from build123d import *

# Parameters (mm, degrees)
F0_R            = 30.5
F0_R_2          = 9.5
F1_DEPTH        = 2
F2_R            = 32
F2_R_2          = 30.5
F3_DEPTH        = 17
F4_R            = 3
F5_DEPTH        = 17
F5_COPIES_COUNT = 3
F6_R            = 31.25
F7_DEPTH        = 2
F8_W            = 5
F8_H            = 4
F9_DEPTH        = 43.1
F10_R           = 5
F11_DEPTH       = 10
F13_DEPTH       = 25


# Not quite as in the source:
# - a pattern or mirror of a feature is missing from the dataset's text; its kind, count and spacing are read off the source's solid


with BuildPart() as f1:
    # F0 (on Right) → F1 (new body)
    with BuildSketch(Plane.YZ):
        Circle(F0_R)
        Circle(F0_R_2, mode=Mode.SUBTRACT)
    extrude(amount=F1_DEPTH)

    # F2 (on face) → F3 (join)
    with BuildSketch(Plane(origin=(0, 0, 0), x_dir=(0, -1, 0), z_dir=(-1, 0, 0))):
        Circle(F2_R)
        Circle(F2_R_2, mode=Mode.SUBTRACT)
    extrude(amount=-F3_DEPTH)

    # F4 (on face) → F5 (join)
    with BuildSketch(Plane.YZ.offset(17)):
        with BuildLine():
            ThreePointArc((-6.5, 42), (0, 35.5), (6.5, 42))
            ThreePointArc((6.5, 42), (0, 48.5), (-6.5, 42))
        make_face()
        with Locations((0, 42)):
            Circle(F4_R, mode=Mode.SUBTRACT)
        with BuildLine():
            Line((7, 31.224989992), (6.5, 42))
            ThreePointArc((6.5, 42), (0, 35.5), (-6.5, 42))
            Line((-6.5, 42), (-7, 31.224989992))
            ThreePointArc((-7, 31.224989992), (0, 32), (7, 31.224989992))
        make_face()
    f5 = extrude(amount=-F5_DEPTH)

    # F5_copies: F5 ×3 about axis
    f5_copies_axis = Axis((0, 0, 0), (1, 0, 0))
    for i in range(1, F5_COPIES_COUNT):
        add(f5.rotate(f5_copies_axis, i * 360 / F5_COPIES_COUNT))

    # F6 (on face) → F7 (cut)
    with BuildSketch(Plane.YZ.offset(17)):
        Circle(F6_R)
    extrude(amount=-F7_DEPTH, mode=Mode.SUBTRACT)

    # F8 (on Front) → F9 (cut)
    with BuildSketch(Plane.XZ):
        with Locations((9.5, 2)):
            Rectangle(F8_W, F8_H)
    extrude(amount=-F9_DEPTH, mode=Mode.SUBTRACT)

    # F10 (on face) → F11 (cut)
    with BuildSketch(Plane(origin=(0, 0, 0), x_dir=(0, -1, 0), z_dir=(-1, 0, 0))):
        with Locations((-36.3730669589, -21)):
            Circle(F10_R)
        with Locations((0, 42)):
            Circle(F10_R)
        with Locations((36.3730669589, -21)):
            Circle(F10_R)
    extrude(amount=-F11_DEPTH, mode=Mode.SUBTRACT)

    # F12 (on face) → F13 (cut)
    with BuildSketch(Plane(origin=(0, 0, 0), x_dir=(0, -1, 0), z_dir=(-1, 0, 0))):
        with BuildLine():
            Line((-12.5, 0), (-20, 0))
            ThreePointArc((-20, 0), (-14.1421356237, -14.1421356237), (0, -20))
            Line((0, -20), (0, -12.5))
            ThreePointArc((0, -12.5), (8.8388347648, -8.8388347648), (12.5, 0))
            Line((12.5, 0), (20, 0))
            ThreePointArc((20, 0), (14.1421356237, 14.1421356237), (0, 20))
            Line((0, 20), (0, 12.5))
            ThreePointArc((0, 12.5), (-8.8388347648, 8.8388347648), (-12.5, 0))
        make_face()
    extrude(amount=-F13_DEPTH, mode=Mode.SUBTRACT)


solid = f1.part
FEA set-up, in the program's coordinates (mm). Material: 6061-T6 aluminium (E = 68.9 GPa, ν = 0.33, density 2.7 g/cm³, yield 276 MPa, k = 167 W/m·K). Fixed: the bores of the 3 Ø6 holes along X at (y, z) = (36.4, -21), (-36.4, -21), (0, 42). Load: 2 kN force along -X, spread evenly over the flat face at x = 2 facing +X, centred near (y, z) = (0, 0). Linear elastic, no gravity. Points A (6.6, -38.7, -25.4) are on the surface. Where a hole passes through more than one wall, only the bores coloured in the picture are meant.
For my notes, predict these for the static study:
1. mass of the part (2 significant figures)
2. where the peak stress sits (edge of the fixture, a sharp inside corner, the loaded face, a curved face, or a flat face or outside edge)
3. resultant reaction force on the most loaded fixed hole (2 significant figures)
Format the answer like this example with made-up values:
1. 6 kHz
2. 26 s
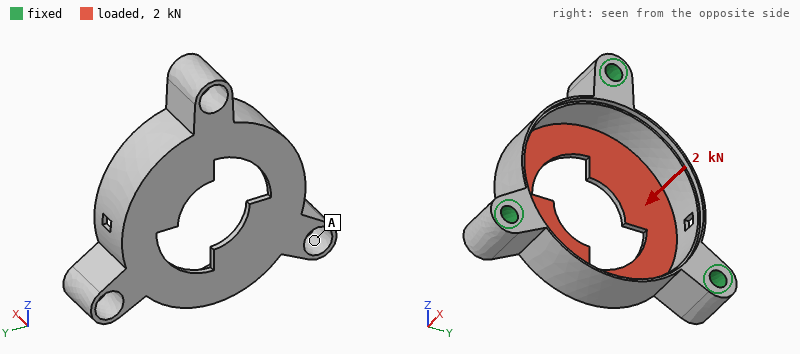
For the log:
1. 44 g
2. a flat face or outside edge
3. 800 N
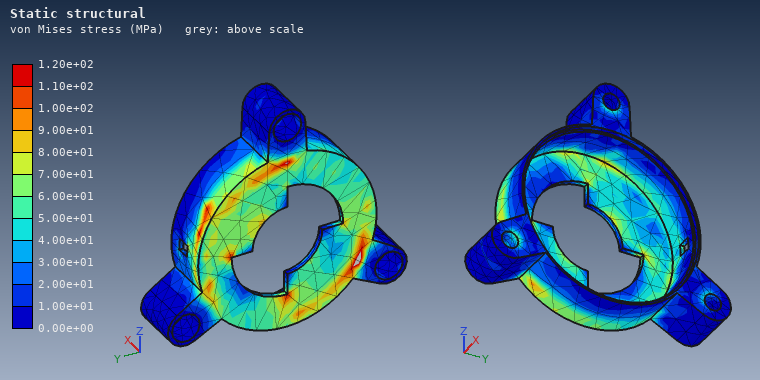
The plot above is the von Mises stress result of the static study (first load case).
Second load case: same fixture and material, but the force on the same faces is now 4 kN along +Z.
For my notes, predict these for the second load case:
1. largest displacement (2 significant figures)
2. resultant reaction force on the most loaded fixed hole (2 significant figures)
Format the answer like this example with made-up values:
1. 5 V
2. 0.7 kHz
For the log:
1. 67 µm
2. 1.5 kN
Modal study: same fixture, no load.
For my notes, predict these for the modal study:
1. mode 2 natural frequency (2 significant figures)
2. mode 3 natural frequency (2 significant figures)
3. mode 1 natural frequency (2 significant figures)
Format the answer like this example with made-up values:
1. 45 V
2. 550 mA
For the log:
1. 6500 Hz
2. 9100 Hz
3. 6200 Hz
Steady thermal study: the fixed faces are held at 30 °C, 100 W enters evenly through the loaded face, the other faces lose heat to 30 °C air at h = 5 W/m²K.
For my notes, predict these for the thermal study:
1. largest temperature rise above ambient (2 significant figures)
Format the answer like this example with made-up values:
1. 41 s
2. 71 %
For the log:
1. 59 K
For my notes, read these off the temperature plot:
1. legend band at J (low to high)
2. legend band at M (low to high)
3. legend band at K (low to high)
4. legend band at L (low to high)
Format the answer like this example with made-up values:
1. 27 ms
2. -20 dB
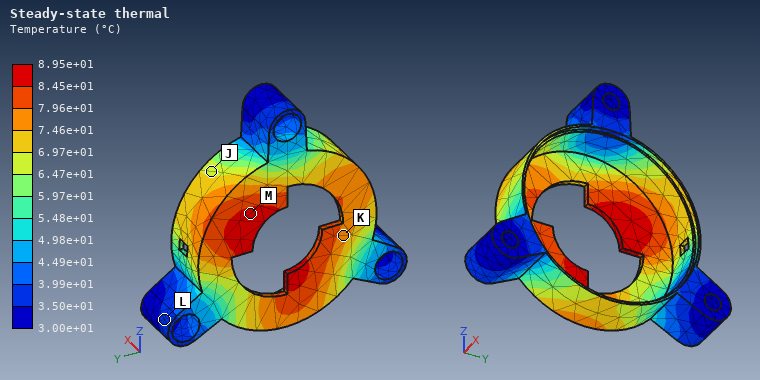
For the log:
1. 6.47e+01 to 6.97e+01 °C
2. 8.45e+01 to 8.95e+01 °C
3. 7.46e+01 to 7.96e+01 °C
4. 3.50e+01 to 3.99e+01 °C
